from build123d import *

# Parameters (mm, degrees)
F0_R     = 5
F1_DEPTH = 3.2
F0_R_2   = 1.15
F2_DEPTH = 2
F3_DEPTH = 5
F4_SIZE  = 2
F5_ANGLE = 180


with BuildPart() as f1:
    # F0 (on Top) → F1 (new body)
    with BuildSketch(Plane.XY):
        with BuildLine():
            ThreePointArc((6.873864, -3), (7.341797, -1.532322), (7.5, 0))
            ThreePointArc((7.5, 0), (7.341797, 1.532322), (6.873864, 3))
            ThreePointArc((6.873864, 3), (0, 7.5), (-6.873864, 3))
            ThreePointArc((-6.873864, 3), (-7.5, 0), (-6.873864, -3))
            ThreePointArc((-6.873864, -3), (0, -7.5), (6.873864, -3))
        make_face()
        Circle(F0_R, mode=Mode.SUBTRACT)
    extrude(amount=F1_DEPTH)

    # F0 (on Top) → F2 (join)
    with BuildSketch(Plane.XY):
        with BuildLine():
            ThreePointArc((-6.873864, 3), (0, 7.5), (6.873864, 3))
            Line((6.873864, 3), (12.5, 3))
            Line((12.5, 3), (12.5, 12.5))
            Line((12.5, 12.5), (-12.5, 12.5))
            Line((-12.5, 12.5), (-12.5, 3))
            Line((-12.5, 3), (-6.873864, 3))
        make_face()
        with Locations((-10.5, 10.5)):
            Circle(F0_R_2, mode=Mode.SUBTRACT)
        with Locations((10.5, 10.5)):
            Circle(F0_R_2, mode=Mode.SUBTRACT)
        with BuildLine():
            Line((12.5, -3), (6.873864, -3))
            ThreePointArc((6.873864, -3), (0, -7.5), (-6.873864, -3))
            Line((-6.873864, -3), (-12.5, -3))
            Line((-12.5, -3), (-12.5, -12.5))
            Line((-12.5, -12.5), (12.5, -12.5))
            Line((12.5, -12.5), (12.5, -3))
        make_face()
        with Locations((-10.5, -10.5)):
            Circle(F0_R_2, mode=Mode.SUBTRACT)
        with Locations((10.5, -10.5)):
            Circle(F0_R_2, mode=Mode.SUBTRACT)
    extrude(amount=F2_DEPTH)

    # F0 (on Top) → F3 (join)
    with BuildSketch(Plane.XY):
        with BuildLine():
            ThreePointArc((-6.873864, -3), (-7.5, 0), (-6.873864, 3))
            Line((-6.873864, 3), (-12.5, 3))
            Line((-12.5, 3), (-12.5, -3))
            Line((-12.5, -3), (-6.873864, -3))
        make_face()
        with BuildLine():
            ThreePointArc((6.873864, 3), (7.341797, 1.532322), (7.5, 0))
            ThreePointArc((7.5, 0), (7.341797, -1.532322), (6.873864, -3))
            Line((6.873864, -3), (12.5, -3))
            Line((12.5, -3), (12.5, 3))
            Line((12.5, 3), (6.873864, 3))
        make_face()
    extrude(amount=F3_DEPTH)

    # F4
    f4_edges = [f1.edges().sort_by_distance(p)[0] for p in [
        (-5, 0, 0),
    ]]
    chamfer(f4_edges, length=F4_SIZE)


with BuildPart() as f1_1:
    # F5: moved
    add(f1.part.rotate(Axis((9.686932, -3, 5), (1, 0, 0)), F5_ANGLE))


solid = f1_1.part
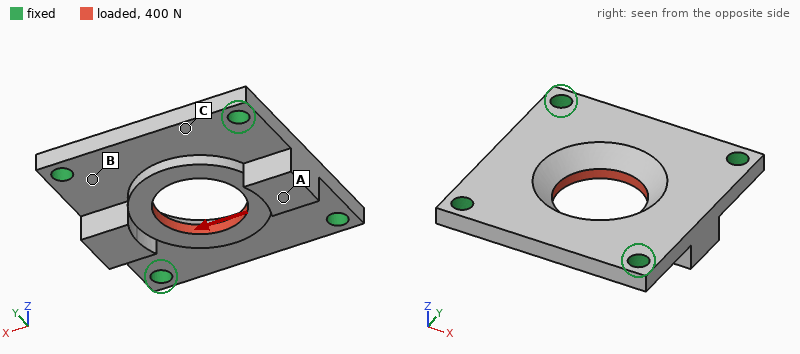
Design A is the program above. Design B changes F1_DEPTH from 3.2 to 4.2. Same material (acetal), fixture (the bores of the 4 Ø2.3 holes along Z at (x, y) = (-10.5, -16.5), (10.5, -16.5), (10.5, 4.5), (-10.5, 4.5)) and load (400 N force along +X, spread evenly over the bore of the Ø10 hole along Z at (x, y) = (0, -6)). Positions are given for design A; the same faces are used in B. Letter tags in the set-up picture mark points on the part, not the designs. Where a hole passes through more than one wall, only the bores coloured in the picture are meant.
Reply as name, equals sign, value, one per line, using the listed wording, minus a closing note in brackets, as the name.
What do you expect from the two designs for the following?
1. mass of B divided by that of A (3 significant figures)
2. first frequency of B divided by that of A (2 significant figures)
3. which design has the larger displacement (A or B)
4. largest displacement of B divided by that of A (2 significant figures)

mass of B divided by that of A = 1.08
first frequency of B divided by that of A = 1.00
which design has the larger displacement = B
largest displacement of B divided by that of A = 1.1
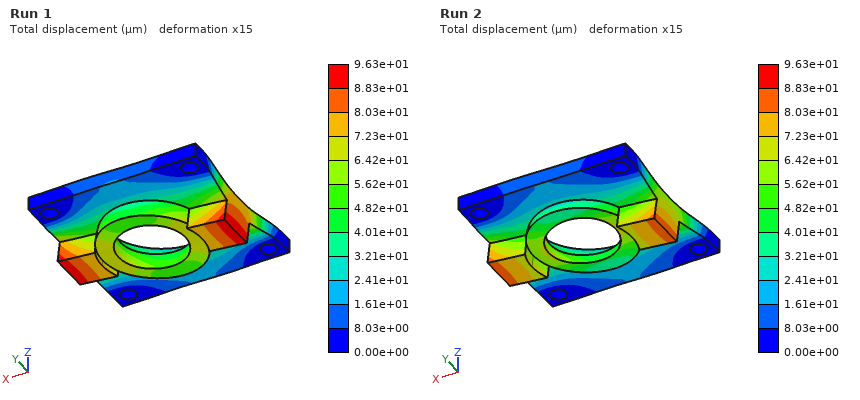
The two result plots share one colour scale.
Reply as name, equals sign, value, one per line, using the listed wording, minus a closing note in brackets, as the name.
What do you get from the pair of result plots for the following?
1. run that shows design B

run that shows design B = Run 1
